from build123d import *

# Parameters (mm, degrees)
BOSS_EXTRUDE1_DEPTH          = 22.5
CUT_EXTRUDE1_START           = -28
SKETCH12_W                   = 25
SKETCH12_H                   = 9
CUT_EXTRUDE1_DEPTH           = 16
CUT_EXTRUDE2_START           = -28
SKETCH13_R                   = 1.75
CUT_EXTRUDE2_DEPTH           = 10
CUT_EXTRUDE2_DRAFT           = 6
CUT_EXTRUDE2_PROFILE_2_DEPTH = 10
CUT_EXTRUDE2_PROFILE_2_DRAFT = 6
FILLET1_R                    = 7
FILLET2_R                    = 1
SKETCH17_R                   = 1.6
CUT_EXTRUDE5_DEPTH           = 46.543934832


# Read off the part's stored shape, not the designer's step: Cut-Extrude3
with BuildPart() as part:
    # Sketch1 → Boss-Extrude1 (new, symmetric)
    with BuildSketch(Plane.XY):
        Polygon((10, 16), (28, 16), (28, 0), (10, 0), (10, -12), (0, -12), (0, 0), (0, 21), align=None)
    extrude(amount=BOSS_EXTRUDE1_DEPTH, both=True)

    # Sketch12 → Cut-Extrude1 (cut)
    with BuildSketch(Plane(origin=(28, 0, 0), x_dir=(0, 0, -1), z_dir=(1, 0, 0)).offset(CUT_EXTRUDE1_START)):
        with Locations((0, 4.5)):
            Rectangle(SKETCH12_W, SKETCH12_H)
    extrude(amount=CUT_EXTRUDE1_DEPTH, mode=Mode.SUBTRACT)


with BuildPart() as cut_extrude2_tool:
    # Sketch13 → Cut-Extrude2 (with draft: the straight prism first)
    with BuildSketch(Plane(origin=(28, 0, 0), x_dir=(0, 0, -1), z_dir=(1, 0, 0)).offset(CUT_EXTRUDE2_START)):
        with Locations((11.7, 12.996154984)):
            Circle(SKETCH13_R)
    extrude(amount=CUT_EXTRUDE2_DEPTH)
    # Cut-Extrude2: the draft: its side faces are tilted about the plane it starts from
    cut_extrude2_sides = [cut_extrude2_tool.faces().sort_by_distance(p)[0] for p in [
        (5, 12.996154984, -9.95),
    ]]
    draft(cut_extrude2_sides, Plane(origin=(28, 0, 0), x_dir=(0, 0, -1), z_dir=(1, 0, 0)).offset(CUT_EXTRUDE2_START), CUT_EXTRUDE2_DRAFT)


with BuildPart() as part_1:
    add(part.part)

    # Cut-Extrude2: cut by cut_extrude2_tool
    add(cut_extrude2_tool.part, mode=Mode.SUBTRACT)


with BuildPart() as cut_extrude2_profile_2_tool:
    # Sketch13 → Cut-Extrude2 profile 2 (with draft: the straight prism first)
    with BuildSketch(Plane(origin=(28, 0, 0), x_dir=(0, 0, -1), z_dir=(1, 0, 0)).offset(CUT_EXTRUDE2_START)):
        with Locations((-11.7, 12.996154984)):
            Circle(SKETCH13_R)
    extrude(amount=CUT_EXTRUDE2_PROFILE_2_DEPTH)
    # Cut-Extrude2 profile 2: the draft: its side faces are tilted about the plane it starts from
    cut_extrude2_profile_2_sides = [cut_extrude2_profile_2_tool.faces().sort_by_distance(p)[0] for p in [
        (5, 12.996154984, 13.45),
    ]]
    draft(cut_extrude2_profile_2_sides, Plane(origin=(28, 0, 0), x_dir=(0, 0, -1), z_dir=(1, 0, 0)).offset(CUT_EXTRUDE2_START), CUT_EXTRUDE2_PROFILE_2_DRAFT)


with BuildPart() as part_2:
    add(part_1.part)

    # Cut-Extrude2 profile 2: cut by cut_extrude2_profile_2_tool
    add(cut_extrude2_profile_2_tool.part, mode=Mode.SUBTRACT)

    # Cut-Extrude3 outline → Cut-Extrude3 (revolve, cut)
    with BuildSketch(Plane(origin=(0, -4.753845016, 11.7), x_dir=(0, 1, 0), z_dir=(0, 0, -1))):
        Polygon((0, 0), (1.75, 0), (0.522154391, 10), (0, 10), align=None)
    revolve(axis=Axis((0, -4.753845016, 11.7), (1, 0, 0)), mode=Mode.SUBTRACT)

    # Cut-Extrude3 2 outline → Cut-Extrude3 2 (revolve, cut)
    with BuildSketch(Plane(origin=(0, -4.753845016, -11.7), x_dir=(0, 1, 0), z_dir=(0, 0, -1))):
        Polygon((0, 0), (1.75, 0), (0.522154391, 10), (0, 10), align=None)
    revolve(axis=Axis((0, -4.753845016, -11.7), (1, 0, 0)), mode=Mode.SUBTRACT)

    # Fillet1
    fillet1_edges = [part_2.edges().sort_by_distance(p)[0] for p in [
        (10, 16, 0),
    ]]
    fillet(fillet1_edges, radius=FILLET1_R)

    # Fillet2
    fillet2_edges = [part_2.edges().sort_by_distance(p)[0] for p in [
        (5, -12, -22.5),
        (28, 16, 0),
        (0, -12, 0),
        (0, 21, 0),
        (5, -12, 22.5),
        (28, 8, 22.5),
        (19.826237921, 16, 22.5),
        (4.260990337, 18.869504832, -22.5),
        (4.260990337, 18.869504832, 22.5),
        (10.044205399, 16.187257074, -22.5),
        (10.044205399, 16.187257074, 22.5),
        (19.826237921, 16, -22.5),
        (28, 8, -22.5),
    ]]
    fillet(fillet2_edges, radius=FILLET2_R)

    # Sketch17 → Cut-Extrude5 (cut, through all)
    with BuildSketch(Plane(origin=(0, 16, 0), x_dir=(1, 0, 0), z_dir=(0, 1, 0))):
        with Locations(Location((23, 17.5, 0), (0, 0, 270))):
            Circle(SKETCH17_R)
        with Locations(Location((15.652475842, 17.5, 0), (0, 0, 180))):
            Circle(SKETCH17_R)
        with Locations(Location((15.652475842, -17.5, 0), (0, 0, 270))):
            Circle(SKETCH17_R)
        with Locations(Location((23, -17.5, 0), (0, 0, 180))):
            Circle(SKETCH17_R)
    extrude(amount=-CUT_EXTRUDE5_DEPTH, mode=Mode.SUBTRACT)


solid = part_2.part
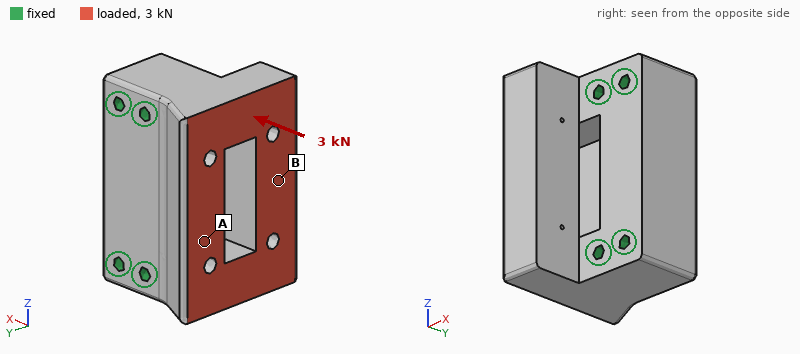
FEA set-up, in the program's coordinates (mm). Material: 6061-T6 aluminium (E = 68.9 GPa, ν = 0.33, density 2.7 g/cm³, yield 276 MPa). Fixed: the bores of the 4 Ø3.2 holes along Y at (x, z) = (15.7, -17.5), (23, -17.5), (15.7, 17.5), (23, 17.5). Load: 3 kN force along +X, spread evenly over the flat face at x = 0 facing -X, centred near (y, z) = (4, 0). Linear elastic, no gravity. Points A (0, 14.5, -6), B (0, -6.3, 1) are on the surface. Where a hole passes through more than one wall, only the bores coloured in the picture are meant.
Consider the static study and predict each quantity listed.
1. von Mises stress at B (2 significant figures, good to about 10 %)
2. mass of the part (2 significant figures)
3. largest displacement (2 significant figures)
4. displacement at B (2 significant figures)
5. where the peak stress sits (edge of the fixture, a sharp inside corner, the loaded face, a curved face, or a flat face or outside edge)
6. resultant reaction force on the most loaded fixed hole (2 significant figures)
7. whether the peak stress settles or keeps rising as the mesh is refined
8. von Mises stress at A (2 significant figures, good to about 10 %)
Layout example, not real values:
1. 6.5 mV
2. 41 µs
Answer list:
1. 11 MPa
2. 60 g
3. 19 µm
4. 15 µm
5. a sharp inside corner
6. 1.2 kN
7. keeps rising
8. 4.2 MPa
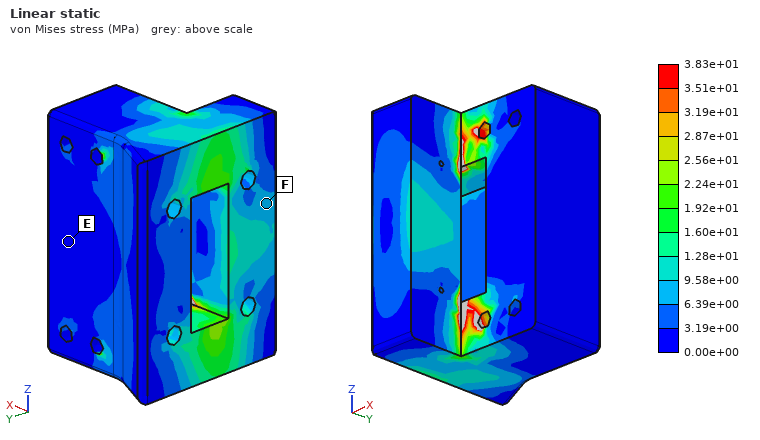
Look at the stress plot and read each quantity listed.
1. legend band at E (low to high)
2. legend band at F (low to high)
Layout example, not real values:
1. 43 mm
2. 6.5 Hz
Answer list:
1. 0.00e+00 to 3.19e+00 MPa
2. 6.39e+00 to 9.58e+00 MPa
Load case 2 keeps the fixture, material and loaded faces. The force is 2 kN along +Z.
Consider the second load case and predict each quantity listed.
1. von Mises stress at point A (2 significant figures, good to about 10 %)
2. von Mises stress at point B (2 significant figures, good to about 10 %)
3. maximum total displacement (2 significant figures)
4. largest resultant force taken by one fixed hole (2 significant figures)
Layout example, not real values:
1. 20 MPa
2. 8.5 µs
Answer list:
1. 4.0 MPa
2. 6.4 MPa
3. 9.0 µm
4. 1.2 kN
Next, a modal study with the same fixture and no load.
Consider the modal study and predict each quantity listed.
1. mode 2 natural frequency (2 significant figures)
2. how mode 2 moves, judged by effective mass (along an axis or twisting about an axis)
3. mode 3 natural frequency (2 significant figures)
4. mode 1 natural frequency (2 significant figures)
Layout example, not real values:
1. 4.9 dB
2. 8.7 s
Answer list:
1. 16 kHz
2. along Z
3. 21 kHz
4. 12 kHz
